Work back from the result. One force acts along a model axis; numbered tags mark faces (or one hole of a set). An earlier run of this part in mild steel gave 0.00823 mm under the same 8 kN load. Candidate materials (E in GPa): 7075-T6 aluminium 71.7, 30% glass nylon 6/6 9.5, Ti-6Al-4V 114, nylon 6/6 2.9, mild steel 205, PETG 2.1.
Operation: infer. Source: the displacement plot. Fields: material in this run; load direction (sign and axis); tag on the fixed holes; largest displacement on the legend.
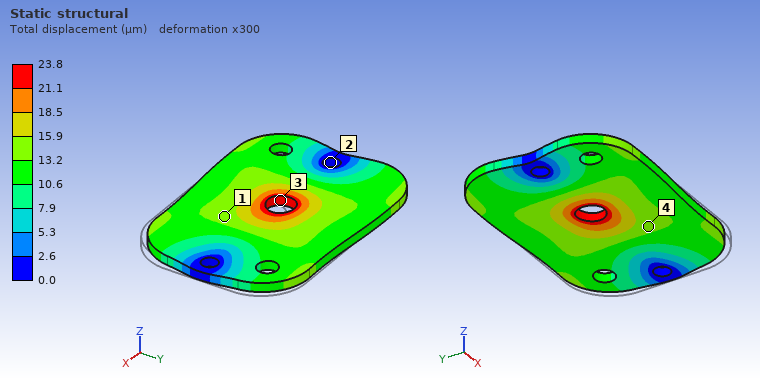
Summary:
7075-T6 aluminium
-X
2
23.8 µm
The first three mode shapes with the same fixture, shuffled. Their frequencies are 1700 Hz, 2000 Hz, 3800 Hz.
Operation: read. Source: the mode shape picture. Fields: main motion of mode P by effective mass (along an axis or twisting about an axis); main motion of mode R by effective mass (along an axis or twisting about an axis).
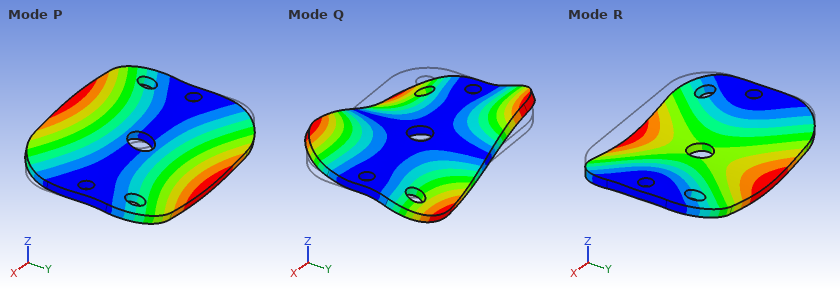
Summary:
twisting about X
along Z
